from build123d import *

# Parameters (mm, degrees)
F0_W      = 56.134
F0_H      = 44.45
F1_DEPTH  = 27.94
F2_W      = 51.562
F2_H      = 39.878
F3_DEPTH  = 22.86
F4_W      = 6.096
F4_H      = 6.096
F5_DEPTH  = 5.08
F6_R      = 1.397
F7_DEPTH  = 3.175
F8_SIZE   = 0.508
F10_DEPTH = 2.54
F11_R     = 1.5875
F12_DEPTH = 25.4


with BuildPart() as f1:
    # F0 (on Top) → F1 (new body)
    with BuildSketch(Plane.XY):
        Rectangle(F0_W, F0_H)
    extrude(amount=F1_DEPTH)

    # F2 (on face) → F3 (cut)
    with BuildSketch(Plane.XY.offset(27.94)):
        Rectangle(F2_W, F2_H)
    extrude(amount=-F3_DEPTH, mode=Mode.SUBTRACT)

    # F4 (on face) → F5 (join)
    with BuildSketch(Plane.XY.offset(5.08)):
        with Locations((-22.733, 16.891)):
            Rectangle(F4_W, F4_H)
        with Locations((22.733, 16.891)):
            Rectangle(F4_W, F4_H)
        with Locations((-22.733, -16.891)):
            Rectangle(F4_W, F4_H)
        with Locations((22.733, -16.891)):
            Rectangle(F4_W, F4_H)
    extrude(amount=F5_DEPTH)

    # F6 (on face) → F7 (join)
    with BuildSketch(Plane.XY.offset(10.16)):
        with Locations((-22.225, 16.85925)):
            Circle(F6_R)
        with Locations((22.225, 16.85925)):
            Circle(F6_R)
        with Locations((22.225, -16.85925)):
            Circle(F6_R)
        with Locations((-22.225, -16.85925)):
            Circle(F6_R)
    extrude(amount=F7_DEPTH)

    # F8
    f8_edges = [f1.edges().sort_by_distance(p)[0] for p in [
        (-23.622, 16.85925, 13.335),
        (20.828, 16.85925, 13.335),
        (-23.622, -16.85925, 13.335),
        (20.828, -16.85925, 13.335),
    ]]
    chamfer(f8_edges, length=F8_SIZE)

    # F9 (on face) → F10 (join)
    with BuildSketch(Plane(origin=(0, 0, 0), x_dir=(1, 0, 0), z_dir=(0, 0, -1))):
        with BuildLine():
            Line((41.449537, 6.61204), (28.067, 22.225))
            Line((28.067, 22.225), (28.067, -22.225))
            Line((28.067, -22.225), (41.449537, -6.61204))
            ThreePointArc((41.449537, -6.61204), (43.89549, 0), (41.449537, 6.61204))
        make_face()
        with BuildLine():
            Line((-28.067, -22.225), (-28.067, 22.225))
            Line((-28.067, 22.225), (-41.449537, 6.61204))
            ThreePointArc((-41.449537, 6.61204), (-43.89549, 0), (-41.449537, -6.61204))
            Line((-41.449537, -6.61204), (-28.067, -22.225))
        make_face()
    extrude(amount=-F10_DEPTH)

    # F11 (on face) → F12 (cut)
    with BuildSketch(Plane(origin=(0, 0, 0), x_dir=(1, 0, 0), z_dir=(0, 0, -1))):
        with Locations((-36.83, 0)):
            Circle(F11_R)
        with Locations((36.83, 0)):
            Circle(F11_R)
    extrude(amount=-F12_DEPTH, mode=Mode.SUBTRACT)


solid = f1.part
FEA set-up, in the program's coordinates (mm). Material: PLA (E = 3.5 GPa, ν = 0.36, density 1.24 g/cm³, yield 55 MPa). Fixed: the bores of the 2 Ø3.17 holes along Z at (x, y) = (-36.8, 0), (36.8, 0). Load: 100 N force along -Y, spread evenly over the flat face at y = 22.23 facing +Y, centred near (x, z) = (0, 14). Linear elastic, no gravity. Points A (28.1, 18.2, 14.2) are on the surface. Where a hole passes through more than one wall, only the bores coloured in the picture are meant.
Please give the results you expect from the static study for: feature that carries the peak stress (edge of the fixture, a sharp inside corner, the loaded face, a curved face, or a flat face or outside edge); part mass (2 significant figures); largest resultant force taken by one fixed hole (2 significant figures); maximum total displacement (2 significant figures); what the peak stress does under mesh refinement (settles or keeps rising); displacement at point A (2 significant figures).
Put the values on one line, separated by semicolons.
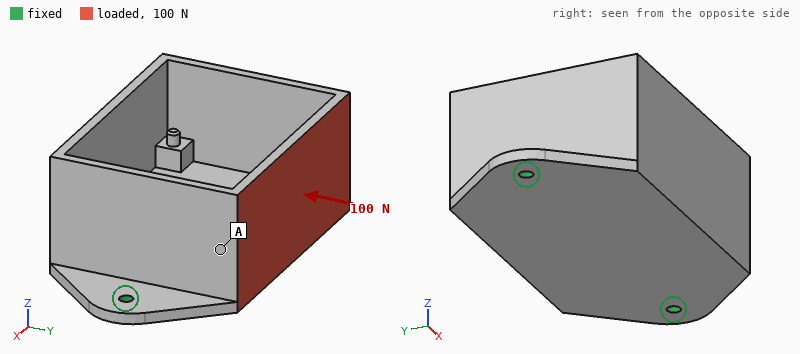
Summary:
edge of the fixture; 32 g; 50 N; 1.2 mm; keeps rising; 0.59 mm
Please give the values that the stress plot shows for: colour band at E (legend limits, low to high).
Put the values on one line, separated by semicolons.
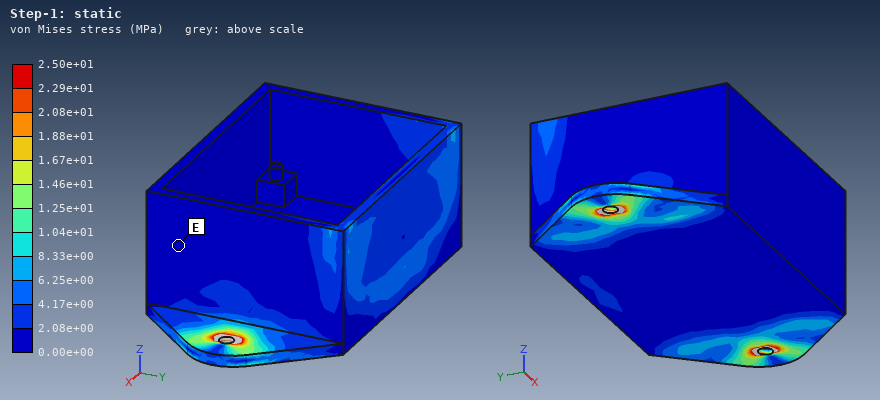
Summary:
0.00e+00 to 2.08e+00 MPa
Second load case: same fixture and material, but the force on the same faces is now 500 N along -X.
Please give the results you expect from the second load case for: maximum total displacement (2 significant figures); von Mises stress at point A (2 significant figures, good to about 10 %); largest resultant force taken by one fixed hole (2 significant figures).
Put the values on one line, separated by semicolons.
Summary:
0.59 mm; 3.8 MPa; 310 N
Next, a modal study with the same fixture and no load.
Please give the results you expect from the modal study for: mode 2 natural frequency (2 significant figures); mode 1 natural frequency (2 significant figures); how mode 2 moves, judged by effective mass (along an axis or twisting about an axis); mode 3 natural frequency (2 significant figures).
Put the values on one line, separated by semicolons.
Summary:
1100 Hz; 340 Hz; along Z; 1200 Hz
